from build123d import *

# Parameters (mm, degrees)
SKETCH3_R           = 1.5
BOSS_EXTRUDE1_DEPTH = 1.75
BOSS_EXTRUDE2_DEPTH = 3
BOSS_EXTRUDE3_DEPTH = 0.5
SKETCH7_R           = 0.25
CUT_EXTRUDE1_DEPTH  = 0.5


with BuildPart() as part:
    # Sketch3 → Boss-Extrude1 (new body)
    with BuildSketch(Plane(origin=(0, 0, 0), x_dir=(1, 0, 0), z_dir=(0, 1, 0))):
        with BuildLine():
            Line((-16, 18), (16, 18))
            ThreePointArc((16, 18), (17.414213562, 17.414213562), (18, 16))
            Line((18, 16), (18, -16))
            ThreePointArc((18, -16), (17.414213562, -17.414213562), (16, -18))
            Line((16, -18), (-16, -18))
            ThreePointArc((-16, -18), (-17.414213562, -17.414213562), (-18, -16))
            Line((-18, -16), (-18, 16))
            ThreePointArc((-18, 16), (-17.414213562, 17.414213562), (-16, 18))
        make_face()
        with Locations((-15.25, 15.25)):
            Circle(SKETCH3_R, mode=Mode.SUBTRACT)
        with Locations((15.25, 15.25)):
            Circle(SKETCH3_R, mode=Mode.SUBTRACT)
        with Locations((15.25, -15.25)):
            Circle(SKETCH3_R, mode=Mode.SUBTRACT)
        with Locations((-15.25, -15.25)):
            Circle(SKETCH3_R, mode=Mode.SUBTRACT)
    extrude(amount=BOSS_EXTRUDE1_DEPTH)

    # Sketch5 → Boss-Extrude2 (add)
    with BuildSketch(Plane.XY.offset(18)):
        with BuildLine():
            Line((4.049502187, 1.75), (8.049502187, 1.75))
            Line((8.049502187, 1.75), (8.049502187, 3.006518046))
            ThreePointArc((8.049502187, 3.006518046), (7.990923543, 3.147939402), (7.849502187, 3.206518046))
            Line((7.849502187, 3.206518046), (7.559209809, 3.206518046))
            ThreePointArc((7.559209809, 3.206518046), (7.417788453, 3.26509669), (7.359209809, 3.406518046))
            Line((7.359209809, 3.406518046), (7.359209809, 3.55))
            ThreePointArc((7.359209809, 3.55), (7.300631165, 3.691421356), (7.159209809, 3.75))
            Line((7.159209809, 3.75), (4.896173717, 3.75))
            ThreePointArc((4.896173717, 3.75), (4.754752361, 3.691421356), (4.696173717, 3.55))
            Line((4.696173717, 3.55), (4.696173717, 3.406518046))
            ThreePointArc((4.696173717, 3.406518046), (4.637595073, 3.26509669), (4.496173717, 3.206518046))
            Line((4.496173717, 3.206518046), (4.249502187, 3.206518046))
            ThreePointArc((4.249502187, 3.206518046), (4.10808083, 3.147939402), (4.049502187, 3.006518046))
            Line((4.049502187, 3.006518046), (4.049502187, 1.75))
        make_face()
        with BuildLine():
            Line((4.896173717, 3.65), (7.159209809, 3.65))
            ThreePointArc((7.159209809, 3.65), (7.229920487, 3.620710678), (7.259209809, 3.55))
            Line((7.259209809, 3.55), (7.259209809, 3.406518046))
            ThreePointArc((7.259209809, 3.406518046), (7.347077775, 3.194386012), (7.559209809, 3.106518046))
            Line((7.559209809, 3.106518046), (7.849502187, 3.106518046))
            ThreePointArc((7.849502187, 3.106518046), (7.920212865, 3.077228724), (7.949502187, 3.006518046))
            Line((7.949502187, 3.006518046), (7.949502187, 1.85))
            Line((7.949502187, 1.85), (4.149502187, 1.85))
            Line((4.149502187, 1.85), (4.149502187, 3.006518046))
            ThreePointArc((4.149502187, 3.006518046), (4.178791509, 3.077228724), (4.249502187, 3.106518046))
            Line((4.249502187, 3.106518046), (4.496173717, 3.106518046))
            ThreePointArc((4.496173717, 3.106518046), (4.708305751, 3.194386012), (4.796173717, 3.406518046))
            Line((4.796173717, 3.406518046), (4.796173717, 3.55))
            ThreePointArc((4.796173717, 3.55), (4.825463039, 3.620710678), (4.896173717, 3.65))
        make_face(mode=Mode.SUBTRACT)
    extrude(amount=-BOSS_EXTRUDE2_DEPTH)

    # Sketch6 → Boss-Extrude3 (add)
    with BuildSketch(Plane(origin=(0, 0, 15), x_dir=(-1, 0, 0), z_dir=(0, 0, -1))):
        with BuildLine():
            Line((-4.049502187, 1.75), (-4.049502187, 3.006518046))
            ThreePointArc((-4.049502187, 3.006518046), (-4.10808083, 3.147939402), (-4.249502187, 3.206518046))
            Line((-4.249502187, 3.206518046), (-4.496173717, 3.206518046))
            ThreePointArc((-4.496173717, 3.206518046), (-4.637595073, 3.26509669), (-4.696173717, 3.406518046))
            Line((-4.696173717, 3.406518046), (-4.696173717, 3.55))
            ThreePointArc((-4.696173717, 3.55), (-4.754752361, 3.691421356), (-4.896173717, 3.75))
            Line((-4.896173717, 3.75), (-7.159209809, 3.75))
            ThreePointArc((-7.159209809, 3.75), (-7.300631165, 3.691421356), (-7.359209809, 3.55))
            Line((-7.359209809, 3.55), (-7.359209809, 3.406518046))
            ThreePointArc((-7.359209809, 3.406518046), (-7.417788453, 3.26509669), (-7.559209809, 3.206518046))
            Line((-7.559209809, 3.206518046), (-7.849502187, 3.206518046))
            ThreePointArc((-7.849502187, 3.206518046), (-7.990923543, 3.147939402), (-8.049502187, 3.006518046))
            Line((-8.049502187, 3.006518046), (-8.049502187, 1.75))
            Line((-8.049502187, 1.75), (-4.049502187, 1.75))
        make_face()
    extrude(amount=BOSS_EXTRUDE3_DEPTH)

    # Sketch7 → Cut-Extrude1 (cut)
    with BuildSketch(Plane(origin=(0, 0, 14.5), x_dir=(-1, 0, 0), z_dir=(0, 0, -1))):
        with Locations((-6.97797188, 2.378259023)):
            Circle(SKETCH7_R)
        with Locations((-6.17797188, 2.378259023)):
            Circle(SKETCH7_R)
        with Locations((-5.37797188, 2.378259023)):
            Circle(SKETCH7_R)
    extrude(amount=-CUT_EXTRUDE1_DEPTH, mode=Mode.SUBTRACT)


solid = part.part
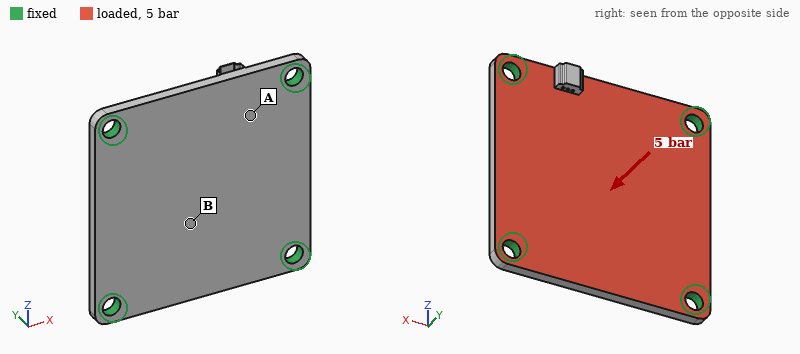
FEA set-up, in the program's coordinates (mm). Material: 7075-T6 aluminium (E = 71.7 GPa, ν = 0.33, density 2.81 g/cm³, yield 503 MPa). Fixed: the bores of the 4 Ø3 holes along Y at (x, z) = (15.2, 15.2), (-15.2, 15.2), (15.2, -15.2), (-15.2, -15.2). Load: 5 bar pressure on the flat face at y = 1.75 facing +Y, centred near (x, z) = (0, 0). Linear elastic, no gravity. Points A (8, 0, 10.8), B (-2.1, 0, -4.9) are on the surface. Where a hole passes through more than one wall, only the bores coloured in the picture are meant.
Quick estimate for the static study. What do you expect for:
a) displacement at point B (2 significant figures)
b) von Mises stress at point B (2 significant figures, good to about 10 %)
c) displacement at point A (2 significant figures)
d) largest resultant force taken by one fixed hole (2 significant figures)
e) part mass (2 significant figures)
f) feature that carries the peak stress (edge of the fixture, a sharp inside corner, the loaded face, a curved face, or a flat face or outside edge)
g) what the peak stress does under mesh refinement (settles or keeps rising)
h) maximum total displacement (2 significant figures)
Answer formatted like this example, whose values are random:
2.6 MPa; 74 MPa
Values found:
71 µm; 42 MPa; 35 µm; 160 N; 6.2 g; edge of the fixture; keeps rising; 78 µm
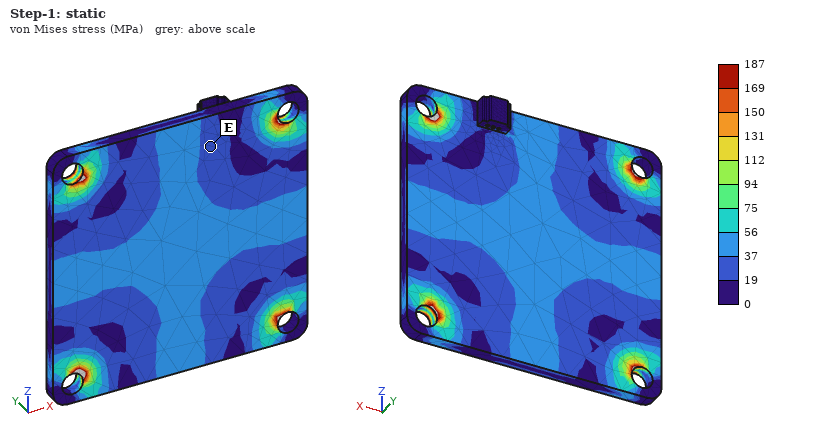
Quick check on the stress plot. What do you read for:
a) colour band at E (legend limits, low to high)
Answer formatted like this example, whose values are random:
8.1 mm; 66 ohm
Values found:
19 to 37 MPa
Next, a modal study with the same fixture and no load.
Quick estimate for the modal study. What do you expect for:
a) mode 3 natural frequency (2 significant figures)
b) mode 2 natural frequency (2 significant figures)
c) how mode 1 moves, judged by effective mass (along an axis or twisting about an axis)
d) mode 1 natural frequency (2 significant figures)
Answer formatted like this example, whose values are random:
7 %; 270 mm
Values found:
12 kHz; 12 kHz; along Y; 7000 Hz
